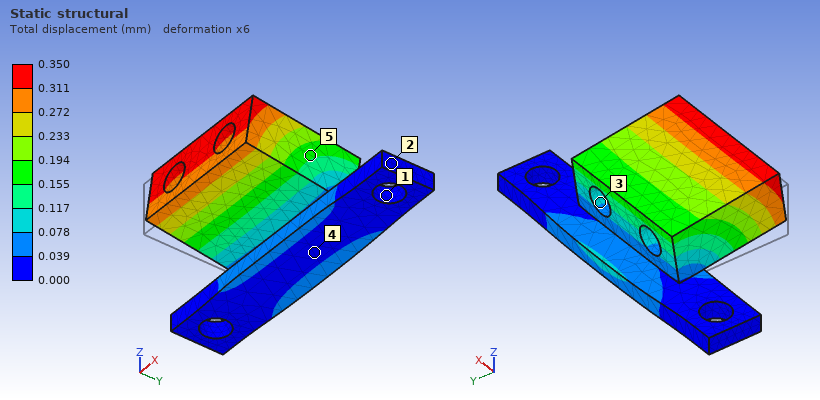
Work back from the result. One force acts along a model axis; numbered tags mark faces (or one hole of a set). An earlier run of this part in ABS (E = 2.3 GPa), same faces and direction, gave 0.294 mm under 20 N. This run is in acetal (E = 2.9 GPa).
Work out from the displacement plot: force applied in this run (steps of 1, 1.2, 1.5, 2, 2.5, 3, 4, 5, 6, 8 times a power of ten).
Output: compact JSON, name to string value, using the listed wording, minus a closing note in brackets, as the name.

{"force applied in this run": "30 N"}
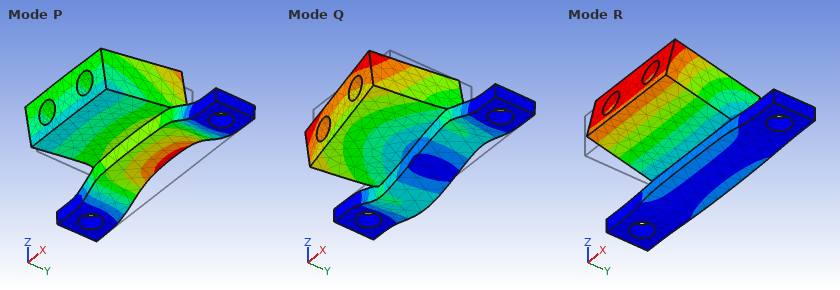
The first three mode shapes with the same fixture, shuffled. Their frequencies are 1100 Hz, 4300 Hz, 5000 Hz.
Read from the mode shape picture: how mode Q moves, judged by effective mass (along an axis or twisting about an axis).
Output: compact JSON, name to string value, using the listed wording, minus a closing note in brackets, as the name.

{"how mode Q moves, judged by effective mass": "along X"}
